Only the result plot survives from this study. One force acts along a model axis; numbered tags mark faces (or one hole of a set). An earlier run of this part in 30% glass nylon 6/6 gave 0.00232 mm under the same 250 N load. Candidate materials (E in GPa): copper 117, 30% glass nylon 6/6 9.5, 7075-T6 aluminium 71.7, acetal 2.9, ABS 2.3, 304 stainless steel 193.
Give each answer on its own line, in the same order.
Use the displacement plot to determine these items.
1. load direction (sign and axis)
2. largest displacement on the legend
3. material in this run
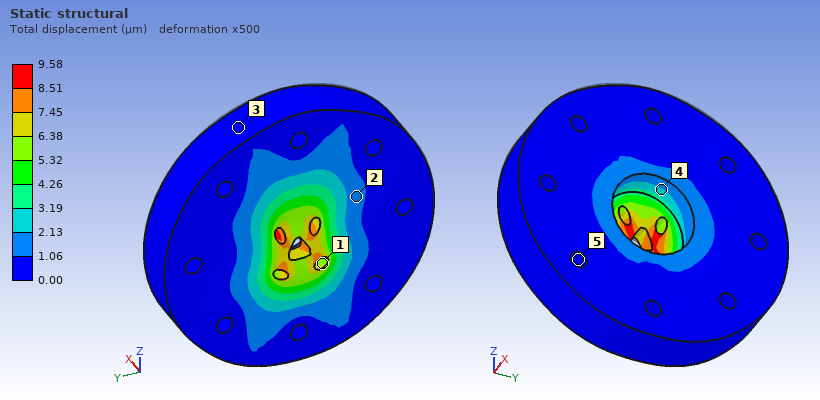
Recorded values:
-Z
9.58 µm
ABS
